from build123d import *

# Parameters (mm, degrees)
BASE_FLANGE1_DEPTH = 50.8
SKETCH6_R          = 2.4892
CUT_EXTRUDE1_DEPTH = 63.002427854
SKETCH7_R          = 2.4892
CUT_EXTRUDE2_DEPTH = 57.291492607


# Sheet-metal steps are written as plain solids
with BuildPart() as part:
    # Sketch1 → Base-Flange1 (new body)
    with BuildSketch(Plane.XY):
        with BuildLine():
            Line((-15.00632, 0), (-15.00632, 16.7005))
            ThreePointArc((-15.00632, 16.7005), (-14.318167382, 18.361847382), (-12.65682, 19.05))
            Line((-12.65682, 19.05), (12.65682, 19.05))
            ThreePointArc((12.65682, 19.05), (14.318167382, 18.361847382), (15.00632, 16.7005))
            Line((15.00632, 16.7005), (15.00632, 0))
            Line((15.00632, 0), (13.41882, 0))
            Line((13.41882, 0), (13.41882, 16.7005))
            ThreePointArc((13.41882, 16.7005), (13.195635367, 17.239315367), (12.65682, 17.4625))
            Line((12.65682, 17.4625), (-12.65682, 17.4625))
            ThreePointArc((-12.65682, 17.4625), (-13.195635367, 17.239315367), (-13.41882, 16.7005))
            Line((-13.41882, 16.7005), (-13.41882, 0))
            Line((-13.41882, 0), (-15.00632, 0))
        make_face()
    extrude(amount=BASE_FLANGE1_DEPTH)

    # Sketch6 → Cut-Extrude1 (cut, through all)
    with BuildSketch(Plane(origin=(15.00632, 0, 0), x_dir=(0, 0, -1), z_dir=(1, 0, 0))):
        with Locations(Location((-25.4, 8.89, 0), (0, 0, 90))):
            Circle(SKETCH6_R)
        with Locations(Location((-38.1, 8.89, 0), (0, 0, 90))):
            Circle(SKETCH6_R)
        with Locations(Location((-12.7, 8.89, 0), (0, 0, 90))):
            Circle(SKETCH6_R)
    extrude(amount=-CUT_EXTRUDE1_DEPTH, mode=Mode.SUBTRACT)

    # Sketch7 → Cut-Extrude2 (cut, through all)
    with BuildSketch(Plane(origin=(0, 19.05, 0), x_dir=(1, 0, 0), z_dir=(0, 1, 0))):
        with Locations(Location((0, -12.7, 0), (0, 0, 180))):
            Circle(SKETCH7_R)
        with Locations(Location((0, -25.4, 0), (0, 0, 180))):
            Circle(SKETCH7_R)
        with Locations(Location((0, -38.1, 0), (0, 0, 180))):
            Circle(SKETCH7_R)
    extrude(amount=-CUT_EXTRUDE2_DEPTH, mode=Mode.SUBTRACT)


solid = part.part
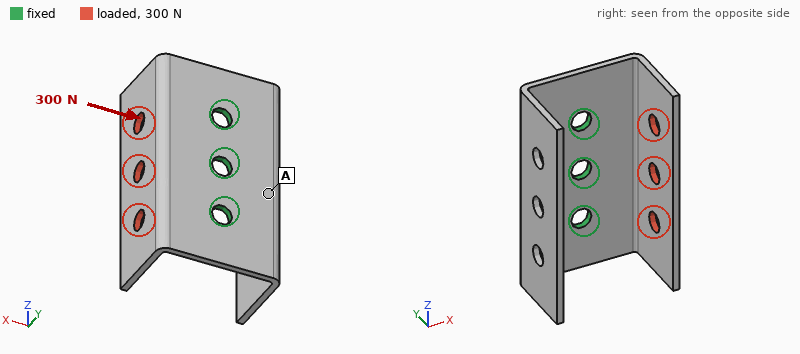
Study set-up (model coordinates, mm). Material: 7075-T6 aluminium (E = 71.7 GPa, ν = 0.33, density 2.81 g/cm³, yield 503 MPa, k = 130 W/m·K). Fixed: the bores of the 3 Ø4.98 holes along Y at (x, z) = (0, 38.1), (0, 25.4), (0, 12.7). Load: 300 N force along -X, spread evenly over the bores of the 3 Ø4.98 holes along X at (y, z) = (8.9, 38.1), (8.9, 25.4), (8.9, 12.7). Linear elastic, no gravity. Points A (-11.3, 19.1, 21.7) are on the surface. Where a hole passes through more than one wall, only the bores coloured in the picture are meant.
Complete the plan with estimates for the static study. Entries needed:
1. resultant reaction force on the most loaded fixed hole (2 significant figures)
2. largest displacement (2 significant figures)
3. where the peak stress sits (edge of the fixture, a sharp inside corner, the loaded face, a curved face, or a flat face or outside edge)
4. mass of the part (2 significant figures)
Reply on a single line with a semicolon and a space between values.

110 N; 0.70 mm; a flat face or outside edge; 14 g
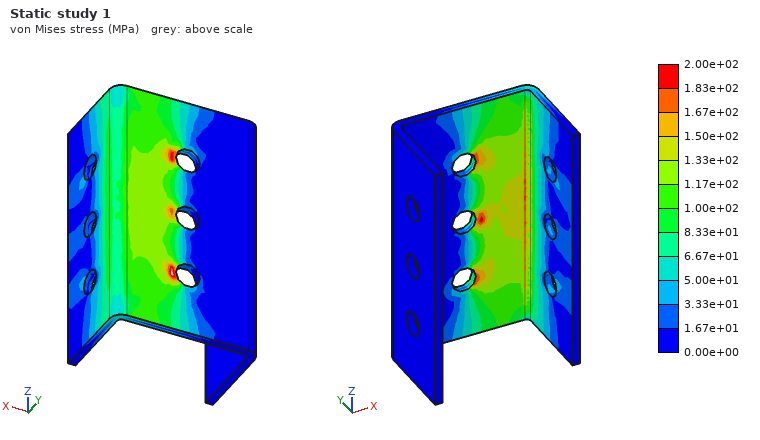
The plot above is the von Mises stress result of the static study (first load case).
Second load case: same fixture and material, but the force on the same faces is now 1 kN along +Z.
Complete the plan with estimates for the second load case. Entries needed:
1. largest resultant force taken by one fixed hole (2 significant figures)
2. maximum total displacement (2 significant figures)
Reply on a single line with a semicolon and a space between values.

640 N; 0.66 mm
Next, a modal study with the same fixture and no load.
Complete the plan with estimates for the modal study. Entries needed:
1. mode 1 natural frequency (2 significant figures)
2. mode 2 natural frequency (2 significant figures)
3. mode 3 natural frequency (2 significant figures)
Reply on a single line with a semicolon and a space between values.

1900 Hz; 1900 Hz; 2600 Hz
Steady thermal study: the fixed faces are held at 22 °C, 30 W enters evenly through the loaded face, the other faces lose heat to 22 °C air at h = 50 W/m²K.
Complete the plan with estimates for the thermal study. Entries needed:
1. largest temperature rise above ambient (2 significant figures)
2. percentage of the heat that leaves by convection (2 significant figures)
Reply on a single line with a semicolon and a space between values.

68 K; 20 %
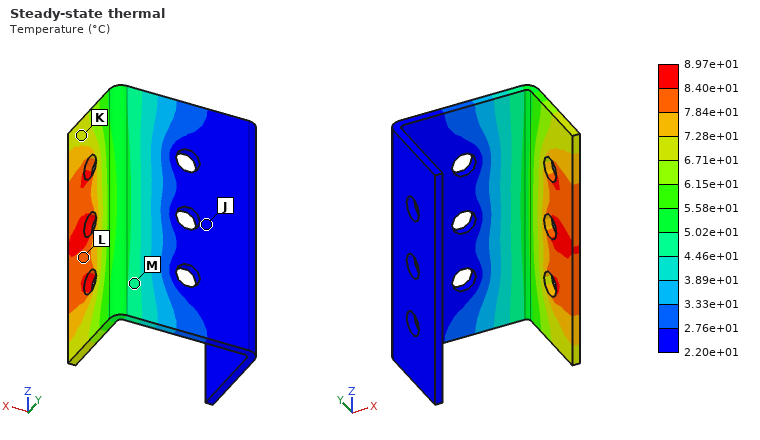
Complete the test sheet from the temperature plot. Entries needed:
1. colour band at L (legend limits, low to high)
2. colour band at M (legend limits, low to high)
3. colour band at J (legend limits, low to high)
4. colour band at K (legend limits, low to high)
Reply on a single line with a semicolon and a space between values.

7.84e+01 to 8.40e+01 °C; 4.46e+01 to 5.02e+01 °C; 2.20e+01 to 2.76e+01 °C; 6.71e+01 to 7.28e+01 °C
